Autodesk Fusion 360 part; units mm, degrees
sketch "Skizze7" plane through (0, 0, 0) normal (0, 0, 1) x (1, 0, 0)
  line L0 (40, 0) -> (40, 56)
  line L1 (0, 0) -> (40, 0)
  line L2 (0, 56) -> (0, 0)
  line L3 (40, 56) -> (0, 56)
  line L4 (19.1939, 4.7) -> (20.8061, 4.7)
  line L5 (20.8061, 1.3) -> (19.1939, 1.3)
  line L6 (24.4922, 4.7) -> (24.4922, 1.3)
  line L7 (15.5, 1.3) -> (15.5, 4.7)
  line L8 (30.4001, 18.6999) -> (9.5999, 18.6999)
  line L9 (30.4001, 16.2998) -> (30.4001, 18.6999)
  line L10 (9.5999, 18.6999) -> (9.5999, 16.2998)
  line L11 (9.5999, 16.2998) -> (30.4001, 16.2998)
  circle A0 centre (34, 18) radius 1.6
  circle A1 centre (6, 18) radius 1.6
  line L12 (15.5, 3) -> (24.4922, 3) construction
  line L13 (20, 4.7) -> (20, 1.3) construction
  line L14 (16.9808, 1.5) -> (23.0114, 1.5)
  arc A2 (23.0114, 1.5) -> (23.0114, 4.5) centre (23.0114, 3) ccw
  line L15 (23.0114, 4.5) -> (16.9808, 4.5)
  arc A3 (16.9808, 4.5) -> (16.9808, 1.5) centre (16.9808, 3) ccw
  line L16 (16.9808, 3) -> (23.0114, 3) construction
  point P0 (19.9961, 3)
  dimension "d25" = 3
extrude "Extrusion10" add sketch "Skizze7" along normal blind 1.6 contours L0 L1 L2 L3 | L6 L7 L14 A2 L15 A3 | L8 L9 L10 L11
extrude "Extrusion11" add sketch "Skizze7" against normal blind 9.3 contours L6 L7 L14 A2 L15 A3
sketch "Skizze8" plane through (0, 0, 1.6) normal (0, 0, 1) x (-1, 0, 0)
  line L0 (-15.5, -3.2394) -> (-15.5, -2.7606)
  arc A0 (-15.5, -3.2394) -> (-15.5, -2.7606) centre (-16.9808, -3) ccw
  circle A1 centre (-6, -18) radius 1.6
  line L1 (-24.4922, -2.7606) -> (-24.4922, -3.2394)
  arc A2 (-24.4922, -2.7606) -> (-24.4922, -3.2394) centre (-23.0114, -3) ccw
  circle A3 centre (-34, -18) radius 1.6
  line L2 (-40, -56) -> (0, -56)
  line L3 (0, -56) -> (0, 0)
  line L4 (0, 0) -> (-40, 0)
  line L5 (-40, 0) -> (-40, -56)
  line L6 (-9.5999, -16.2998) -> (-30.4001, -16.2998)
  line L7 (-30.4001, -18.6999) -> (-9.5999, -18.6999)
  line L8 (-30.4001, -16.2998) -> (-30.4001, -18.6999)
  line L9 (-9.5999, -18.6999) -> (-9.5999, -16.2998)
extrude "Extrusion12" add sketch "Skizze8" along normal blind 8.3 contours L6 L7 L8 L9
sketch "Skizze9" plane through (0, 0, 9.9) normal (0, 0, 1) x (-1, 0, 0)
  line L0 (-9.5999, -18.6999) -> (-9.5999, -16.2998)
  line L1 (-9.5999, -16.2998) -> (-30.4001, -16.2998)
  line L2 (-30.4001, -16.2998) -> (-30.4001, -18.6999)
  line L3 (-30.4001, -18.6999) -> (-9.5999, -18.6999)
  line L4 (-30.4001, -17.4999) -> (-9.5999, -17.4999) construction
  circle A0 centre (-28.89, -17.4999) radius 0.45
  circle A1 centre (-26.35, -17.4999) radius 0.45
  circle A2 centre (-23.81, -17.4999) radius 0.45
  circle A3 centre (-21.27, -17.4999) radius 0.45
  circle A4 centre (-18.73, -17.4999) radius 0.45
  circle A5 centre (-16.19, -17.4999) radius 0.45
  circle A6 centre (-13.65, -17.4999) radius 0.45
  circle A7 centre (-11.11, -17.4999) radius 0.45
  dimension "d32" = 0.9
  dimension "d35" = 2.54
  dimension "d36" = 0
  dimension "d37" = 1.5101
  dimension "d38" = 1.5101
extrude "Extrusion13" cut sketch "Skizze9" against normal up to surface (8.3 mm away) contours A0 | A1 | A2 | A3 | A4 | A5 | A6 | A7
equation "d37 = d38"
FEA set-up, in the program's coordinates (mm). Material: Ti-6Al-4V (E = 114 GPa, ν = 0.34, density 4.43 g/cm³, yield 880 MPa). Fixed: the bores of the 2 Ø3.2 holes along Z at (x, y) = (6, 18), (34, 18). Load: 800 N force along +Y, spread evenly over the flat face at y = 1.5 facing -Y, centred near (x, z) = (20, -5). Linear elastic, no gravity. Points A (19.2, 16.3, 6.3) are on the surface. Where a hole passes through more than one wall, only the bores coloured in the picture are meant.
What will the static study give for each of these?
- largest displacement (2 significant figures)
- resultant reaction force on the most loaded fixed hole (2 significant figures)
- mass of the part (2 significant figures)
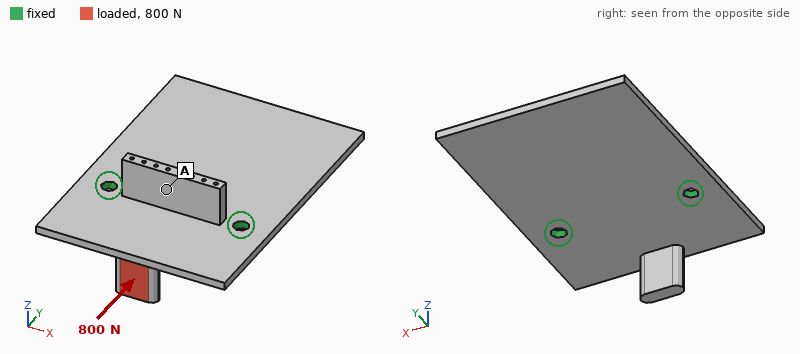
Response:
0.72 mm
420 N
18 g
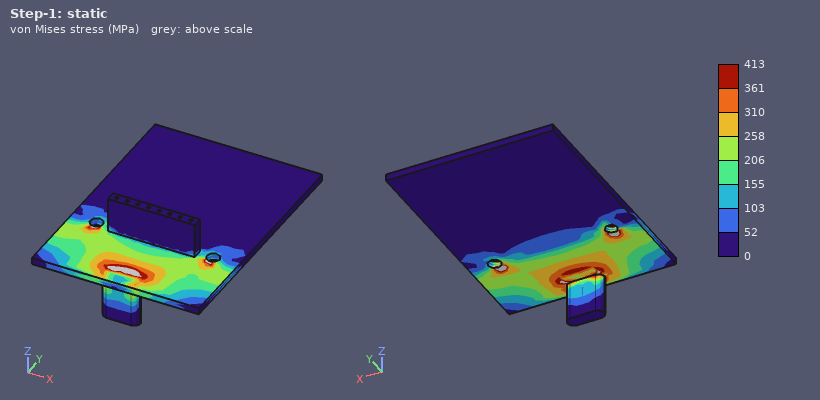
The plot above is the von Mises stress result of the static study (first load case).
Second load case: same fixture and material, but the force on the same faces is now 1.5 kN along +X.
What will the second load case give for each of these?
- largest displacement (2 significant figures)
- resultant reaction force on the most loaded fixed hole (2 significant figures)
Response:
0.42 mm
1.2 kN
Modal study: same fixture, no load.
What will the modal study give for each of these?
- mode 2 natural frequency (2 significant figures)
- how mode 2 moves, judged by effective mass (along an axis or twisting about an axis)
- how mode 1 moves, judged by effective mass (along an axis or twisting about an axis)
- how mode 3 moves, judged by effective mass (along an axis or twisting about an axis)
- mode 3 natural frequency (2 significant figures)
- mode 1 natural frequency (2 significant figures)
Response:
2200 Hz
twisting about Y
along Z
along Z
3100 Hz
920 Hz
